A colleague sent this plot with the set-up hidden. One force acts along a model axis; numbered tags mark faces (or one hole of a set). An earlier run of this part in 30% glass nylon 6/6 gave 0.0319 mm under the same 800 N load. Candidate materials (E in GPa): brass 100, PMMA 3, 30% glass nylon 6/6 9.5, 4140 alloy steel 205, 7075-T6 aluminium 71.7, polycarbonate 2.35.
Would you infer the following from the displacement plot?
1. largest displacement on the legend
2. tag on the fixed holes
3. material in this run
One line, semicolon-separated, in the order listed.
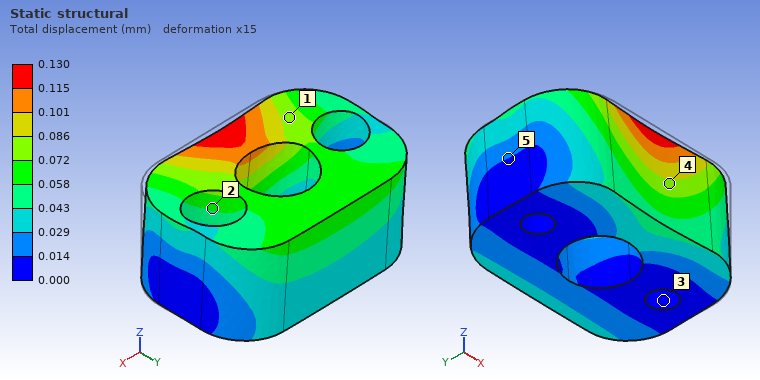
0.130 mm; 3; polycarbonate
